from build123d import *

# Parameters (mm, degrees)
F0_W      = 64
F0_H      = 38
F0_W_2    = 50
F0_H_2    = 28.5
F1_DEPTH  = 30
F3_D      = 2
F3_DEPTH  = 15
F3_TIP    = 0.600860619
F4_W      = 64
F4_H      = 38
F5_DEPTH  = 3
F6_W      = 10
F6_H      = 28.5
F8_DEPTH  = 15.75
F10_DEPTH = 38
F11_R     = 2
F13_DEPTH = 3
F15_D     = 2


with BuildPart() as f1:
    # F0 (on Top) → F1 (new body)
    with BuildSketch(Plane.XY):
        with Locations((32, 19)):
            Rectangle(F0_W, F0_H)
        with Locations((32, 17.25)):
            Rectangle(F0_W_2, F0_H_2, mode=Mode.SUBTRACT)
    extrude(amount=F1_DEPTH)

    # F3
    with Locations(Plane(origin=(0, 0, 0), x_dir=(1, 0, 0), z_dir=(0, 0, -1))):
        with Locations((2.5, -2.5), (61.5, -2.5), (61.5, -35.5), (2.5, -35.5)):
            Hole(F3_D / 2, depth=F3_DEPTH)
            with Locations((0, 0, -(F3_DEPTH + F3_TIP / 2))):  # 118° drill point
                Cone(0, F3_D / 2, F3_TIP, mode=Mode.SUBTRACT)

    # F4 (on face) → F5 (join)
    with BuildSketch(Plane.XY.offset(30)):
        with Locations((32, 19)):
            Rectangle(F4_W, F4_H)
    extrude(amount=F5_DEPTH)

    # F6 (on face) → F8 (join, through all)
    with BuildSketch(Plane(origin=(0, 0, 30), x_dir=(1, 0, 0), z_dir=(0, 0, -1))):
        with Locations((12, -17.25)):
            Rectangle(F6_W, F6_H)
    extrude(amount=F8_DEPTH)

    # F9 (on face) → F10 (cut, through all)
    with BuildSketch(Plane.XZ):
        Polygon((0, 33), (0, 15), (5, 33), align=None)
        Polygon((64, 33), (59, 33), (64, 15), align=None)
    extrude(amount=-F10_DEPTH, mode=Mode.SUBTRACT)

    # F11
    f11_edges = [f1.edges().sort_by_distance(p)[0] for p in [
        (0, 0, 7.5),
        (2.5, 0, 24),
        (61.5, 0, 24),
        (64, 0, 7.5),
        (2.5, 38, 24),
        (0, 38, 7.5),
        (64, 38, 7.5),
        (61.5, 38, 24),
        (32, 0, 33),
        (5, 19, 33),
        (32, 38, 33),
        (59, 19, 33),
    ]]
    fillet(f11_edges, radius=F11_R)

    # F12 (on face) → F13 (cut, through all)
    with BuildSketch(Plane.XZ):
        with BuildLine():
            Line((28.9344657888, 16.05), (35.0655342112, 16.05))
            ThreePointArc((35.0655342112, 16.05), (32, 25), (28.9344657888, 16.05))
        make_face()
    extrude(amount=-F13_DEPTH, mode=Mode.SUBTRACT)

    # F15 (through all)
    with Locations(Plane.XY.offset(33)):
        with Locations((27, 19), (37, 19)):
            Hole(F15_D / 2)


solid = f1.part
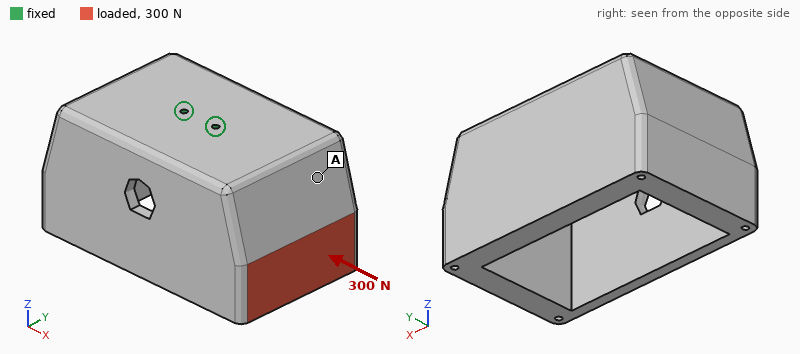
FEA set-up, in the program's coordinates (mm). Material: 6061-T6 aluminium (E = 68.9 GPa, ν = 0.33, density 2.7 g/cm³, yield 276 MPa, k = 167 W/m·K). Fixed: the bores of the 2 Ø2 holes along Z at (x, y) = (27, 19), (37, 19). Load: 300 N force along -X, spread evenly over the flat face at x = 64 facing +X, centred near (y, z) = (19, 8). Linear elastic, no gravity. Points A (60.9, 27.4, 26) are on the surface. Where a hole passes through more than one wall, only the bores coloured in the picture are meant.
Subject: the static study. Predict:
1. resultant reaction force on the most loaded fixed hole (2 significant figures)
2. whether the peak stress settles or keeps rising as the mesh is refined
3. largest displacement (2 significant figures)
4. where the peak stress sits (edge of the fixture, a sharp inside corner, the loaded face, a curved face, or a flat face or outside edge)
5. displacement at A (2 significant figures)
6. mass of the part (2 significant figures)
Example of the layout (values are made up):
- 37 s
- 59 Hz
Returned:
- 500 N
- keeps rising
- 0.11 mm
- edge of the fixture
- 0.073 mm
- 100 g
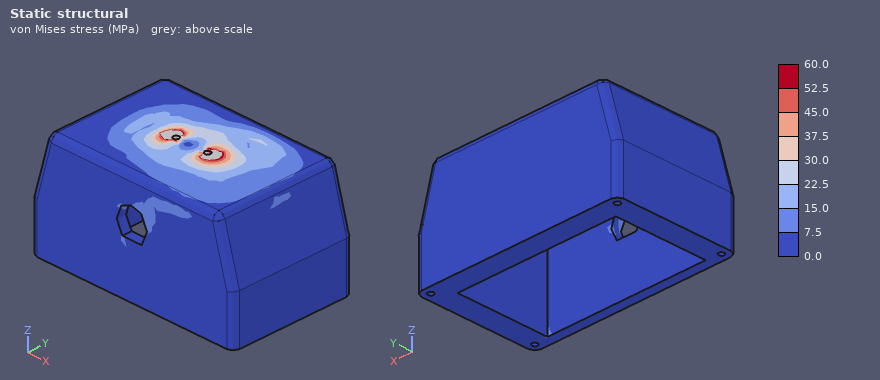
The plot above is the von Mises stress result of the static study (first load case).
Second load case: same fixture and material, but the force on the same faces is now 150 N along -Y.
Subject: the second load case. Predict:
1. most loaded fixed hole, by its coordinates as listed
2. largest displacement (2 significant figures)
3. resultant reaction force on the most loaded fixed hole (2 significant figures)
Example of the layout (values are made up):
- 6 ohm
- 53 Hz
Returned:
- (37, 19)
- 0.12 mm
- 500 N
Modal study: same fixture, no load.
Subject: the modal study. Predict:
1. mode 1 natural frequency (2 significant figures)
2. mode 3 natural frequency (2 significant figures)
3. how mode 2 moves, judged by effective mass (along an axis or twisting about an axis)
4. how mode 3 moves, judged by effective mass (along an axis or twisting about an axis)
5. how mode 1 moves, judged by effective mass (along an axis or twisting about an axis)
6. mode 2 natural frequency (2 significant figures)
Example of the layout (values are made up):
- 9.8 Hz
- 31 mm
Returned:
- 850 Hz
- 2500 Hz
- along X
- twisting about Z
- along Y
- 1000 Hz
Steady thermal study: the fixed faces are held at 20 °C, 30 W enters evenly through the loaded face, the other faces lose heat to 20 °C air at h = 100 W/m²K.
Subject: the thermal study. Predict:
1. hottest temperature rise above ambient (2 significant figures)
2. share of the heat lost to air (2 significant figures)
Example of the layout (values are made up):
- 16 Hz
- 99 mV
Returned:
- 24 K
- 51 %
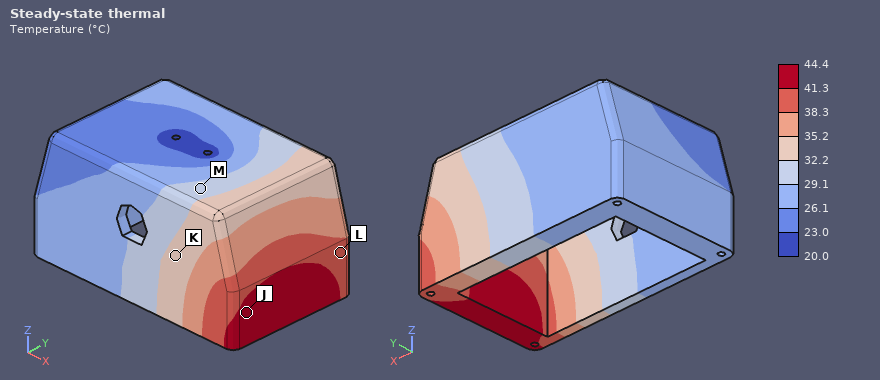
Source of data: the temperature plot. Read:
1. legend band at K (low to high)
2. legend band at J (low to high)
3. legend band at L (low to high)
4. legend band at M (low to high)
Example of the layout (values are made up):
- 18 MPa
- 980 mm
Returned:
- 32.2 to 35.2 °C
- 41.3 to 44.4 °C
- 38.3 to 41.3 °C
- 29.1 to 32.2 °C
